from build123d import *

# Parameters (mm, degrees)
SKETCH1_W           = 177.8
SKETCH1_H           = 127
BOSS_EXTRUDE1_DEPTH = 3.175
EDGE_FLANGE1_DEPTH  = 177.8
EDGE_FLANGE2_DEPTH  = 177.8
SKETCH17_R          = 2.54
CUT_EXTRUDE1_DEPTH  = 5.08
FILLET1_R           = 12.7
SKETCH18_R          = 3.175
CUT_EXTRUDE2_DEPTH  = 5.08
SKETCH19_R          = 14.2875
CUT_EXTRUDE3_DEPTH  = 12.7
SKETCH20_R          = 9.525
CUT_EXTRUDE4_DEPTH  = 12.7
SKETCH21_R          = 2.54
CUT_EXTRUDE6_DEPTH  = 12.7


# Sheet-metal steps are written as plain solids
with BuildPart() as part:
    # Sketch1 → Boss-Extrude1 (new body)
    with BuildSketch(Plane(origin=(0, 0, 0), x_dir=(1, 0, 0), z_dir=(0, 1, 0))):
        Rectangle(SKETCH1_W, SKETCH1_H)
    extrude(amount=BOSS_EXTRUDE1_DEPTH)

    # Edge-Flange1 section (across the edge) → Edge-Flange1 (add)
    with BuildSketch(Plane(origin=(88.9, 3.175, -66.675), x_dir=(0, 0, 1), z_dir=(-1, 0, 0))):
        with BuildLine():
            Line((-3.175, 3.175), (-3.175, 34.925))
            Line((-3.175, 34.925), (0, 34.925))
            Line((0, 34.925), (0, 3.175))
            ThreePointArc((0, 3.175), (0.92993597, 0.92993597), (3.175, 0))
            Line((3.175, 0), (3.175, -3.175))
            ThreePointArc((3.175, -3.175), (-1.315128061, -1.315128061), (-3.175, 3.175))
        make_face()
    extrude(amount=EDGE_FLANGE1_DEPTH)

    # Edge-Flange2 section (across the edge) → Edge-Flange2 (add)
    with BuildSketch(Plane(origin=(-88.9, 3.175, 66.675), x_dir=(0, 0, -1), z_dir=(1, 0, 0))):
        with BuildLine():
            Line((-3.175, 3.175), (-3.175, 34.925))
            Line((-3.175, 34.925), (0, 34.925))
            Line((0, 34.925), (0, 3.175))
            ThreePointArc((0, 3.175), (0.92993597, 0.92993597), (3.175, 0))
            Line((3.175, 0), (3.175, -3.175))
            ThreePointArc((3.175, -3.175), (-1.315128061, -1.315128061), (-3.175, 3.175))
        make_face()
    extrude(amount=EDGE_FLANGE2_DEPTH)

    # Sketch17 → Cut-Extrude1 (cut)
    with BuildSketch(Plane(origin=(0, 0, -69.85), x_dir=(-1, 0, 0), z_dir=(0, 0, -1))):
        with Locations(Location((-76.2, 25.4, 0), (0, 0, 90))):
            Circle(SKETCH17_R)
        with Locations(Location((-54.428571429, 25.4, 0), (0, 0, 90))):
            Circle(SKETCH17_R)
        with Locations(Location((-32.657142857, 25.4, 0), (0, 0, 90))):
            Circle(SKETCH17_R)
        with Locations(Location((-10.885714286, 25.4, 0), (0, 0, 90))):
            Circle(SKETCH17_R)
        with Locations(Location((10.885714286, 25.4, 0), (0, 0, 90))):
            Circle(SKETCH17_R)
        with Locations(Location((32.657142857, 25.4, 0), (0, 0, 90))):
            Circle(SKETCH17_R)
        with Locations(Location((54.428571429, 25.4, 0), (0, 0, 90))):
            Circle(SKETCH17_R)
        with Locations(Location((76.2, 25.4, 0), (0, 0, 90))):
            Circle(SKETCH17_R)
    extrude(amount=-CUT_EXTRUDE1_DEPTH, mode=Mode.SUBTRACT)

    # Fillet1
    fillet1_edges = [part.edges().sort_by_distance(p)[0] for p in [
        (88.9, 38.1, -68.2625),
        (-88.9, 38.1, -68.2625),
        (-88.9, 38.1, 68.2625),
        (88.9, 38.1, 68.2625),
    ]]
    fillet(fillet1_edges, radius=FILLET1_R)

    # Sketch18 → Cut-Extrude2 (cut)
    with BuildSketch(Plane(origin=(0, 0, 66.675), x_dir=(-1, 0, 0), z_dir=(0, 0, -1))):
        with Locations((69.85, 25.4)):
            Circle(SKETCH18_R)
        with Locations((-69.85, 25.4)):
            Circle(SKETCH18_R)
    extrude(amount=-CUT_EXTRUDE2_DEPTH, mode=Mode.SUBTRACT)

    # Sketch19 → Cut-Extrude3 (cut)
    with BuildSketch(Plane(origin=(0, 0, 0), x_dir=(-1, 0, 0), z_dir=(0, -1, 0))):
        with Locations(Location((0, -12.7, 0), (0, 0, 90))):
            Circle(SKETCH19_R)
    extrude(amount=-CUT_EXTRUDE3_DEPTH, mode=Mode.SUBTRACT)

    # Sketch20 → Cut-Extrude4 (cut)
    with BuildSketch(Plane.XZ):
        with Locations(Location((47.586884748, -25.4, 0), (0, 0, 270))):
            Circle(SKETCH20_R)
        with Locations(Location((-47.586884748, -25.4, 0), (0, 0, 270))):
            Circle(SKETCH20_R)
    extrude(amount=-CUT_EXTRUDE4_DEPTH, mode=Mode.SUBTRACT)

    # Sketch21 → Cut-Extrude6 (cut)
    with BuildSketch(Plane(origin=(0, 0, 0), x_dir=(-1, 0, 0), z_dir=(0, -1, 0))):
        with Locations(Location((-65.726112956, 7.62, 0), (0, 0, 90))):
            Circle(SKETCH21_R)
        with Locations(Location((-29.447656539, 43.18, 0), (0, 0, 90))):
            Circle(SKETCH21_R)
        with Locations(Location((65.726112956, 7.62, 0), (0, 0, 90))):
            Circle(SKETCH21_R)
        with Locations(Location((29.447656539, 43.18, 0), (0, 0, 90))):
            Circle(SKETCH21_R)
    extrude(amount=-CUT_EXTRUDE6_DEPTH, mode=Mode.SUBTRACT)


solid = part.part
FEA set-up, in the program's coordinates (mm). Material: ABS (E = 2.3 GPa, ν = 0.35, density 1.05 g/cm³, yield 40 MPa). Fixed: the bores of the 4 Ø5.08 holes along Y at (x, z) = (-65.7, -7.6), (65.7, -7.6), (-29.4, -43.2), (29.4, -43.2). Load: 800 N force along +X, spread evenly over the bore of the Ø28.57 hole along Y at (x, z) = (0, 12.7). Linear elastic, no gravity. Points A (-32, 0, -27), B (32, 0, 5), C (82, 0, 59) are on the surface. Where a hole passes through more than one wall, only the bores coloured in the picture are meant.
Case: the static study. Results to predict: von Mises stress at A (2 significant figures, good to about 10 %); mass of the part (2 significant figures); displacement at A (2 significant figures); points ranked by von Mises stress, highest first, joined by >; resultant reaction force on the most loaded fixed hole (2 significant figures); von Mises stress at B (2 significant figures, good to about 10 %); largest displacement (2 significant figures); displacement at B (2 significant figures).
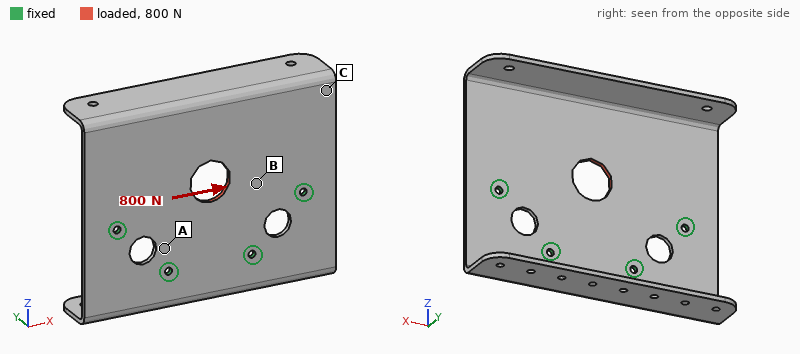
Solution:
1.3 MPa
120 g
0.022 mm
B > A > C
330 N
3.1 MPa
0.12 mm
0.060 mm
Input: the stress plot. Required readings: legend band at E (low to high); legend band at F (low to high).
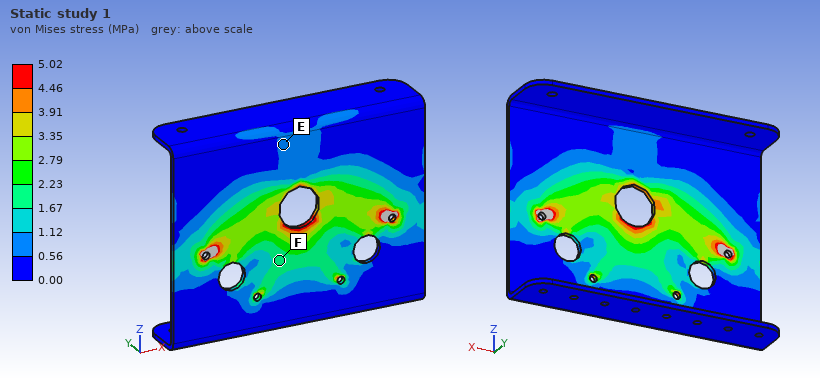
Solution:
0.56 to 1.12 MPa
1.67 to 2.23 MPa
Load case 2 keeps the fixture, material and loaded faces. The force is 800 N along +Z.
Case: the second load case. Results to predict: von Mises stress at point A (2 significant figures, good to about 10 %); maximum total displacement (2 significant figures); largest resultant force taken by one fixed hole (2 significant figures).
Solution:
2.4 MPa
0.10 mm
260 N
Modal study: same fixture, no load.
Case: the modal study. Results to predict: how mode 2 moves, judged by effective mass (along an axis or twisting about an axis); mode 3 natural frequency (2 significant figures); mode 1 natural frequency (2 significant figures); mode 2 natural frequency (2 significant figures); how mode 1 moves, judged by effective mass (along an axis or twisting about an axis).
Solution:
twisting about Z
230 Hz
65 Hz
120 Hz
along Y
